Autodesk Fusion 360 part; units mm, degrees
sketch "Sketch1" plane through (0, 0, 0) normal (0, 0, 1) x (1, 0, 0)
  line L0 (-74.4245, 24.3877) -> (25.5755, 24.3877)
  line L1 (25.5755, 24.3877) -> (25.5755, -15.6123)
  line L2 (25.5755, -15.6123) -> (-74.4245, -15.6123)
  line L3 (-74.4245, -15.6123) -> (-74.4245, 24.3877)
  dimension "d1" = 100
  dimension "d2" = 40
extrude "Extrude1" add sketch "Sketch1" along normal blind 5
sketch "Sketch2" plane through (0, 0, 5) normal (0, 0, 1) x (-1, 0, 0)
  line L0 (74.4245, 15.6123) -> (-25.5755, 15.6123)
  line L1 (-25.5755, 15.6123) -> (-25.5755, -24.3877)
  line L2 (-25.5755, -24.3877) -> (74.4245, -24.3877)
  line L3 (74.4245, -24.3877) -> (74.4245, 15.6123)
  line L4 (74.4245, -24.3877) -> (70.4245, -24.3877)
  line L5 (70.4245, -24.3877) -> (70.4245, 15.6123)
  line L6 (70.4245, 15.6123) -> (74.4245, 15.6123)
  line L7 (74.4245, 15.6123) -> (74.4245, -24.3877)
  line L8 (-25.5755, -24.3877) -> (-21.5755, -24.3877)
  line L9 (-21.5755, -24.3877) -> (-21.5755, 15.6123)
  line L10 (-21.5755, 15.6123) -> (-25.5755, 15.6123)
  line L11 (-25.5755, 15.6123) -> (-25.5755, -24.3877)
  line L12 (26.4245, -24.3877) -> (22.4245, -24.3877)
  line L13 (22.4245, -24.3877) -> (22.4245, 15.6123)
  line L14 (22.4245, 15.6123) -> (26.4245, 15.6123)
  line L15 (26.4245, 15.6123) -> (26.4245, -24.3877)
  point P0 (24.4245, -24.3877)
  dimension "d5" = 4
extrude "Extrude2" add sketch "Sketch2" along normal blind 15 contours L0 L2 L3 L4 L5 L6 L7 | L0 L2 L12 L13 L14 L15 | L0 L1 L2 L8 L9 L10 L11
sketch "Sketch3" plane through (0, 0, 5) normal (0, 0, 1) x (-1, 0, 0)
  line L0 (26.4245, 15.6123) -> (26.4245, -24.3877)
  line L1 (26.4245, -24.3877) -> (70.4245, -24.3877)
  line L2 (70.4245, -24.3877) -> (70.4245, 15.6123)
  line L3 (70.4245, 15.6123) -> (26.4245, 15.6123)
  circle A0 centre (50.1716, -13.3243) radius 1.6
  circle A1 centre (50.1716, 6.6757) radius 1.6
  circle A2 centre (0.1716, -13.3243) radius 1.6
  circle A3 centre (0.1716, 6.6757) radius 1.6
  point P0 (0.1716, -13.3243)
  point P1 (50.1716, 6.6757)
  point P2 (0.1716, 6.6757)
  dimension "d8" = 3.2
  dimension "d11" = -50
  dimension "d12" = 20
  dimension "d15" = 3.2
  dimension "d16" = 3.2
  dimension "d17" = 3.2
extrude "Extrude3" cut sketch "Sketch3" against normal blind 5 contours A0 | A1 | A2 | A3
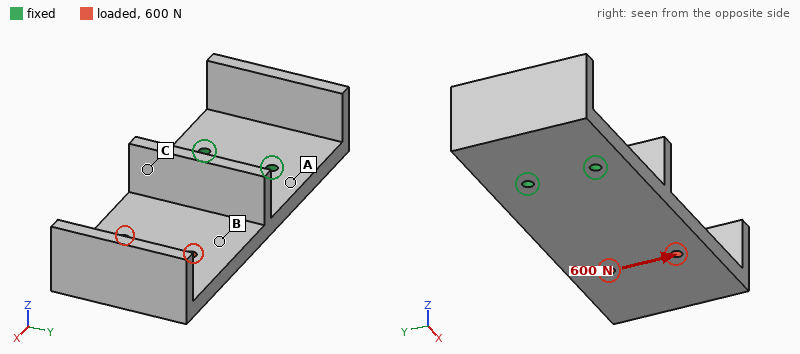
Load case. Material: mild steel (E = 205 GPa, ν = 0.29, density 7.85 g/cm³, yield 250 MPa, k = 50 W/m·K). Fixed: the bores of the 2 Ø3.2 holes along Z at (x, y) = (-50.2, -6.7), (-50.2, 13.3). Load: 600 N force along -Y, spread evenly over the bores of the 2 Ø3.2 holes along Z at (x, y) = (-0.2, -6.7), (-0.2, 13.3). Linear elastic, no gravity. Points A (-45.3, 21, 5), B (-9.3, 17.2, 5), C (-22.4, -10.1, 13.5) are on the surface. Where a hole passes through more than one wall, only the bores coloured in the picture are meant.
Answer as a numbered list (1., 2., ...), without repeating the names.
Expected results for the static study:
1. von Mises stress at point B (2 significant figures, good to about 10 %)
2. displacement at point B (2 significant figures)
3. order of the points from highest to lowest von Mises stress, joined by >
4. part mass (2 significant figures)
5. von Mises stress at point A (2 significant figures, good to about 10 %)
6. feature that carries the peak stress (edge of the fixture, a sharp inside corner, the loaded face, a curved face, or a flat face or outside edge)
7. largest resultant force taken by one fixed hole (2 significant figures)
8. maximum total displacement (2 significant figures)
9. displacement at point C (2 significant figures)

1. 5.5 MPa
2. 7.6 µm
3. A > B > C
4. 210 g
5. 12 MPa
6. edge of the fixture
7. 1.4 kN
8. 15 µm
9. 4.8 µm
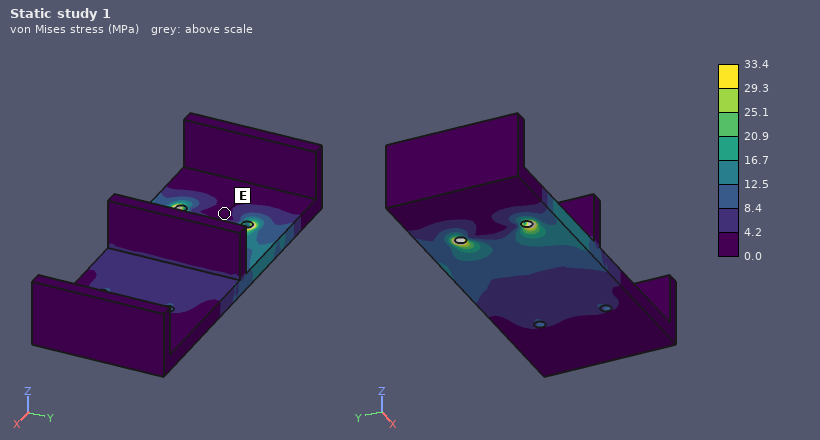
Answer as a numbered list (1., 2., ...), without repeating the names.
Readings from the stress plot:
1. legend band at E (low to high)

1. 0.0 to 4.2 MPa
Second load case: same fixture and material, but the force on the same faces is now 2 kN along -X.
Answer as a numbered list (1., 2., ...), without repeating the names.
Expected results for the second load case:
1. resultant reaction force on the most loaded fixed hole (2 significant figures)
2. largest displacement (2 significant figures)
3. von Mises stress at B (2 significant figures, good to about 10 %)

1. 1.0 kN
2. 3.4 µm
3. 10 MPa
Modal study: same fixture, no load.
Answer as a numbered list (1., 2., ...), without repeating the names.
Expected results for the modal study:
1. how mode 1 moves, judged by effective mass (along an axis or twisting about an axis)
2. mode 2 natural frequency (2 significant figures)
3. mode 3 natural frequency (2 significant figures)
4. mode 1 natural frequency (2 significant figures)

1. along Z
2. 2100 Hz
3. 3100 Hz
4. 560 Hz
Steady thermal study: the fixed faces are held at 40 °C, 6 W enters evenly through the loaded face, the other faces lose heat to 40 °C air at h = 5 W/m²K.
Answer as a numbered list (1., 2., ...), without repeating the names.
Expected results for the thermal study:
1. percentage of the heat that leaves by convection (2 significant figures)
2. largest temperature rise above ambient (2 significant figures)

1. 15 %
2. 29 K
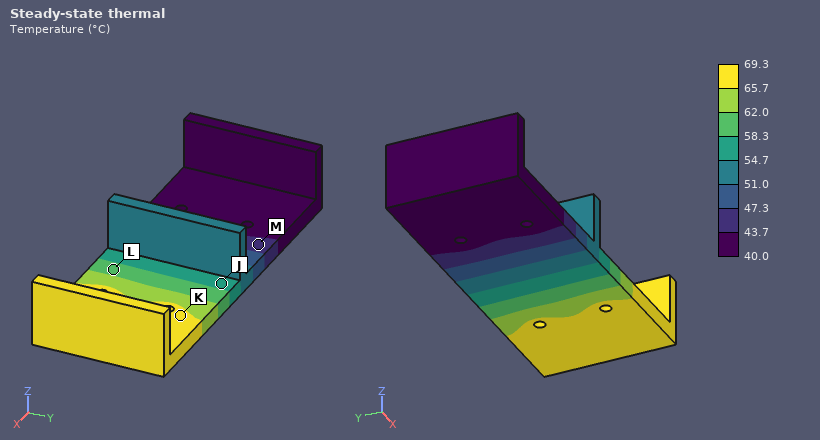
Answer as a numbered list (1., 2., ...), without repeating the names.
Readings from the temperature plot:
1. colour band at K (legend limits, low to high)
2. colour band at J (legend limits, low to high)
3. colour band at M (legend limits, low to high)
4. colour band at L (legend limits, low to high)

1. 65.7 to 69.3 °C
2. 54.7 to 58.3 °C
3. 43.7 to 47.3 °C
4. 58.3 to 62.0 °C
